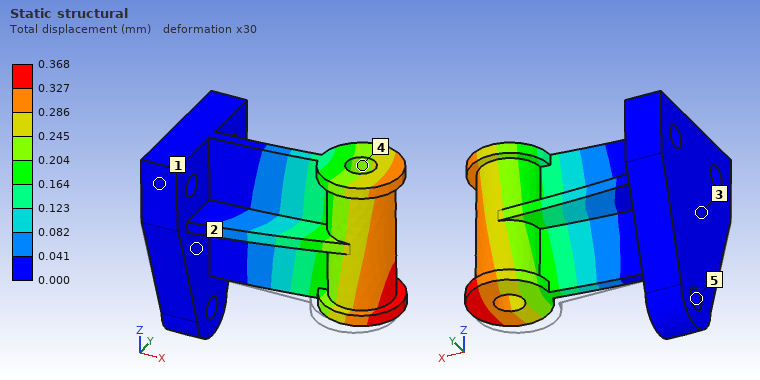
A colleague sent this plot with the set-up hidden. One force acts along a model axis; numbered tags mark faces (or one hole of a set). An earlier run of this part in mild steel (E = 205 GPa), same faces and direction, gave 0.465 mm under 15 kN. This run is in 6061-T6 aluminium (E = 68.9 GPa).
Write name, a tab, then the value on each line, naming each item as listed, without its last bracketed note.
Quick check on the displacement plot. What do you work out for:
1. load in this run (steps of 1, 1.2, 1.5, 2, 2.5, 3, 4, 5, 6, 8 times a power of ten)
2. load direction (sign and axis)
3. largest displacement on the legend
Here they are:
load in this run	4 kN
load direction	+Y
largest displacement on the legend	0.368 mm
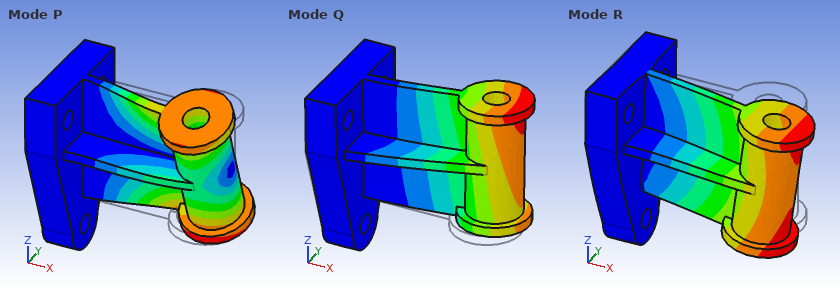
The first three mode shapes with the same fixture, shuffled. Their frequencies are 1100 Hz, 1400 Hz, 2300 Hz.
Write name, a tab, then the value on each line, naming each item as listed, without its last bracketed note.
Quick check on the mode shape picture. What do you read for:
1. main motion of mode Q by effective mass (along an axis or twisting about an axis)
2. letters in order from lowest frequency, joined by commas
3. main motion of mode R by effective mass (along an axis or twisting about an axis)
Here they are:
main motion of mode Q by effective mass	along Y
letters in order from lowest frequency, joined by commas	P, Q, R
main motion of mode R by effective mass	along Z
